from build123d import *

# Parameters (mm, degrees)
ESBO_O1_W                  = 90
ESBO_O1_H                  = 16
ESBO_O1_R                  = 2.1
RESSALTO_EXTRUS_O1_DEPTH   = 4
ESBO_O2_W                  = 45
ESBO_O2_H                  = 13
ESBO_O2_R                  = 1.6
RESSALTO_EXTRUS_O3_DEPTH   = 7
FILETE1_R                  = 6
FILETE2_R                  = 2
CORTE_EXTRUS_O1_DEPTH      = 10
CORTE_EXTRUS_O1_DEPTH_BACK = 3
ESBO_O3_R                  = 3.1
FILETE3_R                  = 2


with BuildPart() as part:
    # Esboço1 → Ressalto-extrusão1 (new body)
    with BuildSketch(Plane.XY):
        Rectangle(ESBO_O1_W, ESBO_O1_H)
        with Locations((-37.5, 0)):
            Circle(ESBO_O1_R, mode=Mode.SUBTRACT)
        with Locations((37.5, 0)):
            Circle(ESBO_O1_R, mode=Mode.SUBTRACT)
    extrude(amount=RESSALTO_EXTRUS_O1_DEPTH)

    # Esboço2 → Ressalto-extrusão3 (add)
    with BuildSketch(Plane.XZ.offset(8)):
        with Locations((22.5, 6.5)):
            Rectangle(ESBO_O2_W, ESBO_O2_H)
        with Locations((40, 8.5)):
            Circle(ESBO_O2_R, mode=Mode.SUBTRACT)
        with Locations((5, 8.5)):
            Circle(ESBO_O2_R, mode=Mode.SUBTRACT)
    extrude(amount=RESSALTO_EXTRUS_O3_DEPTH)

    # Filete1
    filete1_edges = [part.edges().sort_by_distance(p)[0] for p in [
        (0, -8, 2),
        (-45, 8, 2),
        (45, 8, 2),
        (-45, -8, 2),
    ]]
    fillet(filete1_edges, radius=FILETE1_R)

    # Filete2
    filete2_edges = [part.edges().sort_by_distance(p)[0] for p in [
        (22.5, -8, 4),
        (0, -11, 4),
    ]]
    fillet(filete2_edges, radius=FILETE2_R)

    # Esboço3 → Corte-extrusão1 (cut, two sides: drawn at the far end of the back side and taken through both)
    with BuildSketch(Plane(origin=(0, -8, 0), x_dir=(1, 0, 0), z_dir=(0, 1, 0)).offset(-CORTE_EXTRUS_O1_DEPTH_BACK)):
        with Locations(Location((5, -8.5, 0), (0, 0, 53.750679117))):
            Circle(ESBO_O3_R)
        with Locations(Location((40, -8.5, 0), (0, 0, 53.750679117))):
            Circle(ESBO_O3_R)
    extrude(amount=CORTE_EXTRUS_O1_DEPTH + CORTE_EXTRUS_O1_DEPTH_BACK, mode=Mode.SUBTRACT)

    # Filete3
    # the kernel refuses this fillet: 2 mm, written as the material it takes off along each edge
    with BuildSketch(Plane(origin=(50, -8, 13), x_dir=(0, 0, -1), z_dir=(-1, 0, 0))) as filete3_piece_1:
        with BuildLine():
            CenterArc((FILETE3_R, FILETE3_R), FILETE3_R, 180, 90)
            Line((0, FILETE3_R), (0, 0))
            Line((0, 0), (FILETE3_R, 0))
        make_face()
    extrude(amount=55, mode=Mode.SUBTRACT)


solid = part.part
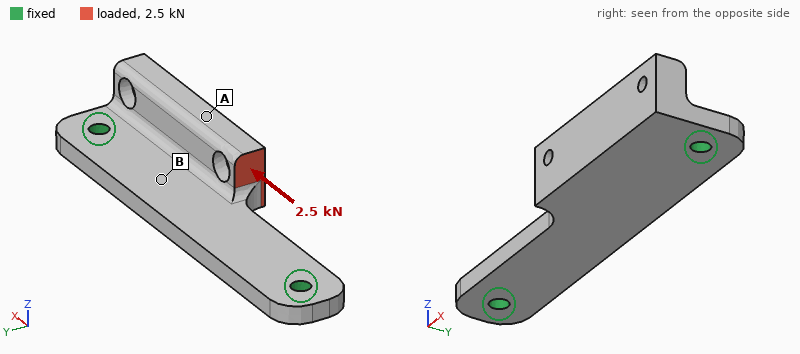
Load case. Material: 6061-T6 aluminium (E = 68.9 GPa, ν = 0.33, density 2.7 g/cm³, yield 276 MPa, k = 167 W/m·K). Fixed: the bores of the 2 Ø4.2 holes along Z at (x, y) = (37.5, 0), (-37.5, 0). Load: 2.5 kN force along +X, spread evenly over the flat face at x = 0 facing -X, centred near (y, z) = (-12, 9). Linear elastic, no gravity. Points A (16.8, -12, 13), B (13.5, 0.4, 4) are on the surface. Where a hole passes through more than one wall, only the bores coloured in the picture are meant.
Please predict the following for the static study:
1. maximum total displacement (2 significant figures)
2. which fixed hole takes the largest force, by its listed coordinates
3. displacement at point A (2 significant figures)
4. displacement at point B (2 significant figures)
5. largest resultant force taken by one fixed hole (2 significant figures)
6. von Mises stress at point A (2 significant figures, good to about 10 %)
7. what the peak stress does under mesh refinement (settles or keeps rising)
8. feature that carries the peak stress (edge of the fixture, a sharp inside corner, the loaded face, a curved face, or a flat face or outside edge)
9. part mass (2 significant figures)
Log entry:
0.18 mm
(37.5, 0)
0.10 mm
0.073 mm
1.8 kN
38 MPa
keeps rising
edge of the fixture
25 g
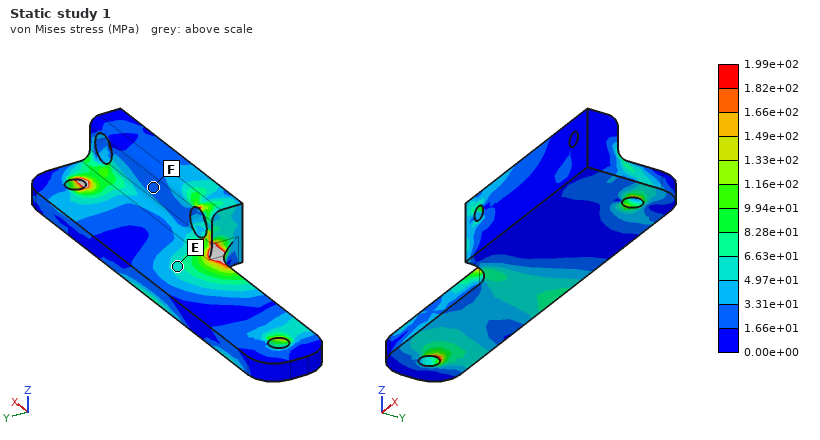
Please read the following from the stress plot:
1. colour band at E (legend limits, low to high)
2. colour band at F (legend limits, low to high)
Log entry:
4.97e+01 to 6.63e+01 MPa
1.66e+01 to 3.31e+01 MPa
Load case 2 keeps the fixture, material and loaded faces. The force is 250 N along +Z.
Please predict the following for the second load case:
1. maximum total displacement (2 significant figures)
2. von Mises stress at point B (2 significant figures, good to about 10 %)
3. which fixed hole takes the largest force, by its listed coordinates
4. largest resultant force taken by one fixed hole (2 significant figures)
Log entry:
0.13 mm
9.6 MPa
(37.5, 0)
140 N
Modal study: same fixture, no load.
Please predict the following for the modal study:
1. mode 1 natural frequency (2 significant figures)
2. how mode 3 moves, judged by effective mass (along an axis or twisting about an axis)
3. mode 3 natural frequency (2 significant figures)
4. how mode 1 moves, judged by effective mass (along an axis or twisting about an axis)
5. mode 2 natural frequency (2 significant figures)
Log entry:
3100 Hz
along Y
7900 Hz
along Z
5100 Hz
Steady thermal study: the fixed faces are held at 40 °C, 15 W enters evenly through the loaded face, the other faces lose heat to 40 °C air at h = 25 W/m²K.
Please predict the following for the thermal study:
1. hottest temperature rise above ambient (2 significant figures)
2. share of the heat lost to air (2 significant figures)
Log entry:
32 K
7.5 %
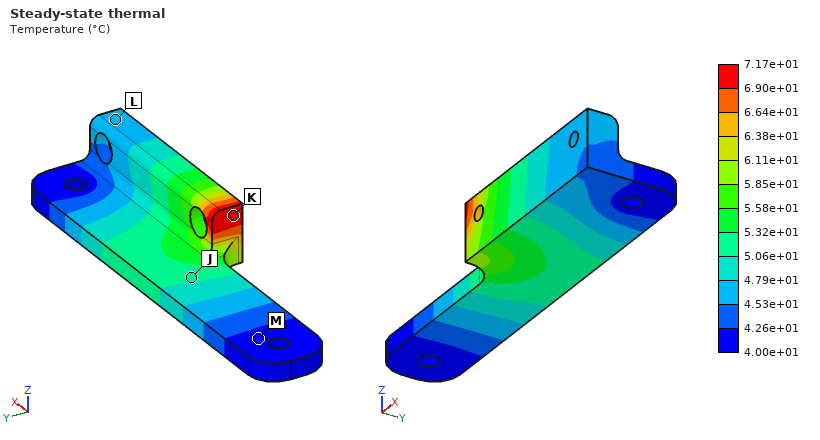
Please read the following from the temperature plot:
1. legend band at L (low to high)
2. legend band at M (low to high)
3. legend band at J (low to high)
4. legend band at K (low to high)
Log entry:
4.53e+01 to 4.79e+01 °C
4.00e+01 to 4.26e+01 °C
5.06e+01 to 5.32e+01 °C
6.90e+01 to 7.17e+01 °C
